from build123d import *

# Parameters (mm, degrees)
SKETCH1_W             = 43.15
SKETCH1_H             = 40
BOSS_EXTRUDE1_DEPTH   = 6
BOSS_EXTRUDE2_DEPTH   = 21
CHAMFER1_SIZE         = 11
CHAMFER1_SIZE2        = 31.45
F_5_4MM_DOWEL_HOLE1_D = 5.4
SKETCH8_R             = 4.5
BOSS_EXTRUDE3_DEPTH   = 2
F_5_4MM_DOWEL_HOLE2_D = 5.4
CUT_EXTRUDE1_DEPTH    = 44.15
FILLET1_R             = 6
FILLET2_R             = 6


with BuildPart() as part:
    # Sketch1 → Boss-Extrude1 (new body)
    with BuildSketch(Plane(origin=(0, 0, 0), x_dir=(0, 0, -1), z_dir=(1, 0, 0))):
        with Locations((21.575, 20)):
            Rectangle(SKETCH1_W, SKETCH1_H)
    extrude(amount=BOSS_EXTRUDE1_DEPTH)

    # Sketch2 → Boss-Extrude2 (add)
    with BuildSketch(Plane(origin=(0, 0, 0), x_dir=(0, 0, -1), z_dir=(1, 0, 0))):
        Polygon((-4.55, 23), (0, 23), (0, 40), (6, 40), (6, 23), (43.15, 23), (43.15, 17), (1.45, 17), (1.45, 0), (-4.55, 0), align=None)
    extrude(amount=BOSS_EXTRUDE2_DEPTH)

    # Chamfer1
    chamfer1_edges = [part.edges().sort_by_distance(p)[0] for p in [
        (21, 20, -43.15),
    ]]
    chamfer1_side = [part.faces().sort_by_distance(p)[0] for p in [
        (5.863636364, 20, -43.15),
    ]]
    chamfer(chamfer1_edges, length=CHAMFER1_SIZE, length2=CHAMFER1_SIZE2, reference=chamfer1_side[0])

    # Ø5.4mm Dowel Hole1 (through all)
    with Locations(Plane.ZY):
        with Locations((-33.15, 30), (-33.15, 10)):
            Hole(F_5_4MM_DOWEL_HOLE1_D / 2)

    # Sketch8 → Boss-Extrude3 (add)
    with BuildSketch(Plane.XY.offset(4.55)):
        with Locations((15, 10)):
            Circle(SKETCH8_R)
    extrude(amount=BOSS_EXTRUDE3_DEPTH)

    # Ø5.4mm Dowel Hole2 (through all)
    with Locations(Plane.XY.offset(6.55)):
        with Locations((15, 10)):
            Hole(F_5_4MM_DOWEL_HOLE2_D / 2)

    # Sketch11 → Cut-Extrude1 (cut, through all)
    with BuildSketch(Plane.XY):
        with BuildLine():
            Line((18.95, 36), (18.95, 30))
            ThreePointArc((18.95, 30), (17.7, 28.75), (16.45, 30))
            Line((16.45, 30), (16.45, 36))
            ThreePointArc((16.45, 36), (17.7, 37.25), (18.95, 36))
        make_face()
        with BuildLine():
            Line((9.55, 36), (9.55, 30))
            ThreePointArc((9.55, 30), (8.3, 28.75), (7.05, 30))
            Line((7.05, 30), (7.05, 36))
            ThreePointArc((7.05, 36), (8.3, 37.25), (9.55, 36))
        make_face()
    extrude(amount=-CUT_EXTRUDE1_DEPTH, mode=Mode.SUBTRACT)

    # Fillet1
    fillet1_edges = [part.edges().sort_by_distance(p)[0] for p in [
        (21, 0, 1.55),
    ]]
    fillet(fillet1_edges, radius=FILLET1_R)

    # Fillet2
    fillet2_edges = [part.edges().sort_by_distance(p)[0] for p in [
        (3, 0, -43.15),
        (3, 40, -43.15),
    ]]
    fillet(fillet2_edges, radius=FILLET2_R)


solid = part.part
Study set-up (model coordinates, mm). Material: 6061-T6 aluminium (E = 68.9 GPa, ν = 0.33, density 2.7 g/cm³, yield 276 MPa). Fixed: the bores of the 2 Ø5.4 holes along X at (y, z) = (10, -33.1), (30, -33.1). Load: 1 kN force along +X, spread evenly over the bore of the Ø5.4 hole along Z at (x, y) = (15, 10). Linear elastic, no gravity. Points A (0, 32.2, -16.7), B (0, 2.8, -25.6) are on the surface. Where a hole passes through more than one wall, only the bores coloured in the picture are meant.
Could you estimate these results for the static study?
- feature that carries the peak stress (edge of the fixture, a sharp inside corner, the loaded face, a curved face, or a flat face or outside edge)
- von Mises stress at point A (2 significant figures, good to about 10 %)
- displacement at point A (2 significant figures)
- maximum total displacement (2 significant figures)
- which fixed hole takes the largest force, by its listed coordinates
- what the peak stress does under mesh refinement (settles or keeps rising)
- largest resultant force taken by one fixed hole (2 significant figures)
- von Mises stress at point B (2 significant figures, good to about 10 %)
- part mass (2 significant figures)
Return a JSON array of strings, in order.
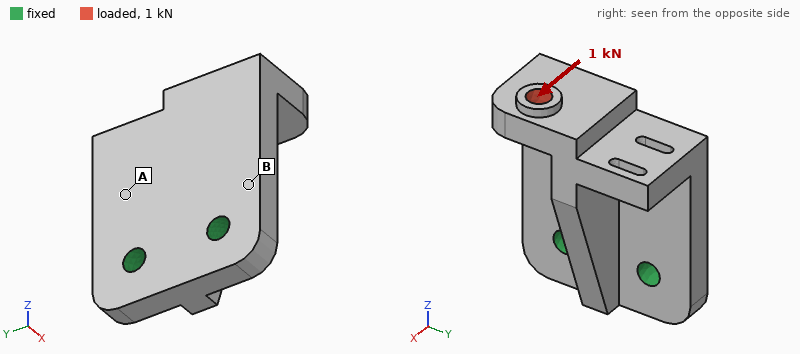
["edge of the fixture", "27 MPa", "0.036 mm", "0.20 mm", "(10, -33.1)", "keeps rising", "970 N", "64 MPa", "45 g"]
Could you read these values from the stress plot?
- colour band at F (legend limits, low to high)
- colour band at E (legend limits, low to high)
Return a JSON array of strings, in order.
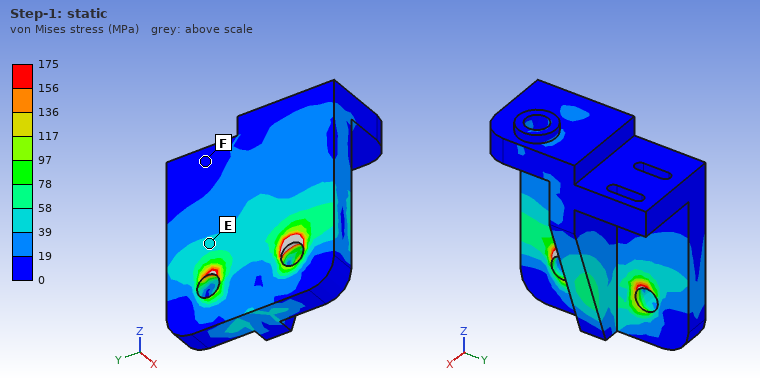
["0 to 19 MPa", "39 to 58 MPa"]
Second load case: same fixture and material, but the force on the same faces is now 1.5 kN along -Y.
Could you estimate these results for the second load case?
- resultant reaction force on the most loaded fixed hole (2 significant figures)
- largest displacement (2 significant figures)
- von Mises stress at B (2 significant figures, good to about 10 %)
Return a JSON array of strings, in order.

["2.5 kN", "0.10 mm", "42 MPa"]
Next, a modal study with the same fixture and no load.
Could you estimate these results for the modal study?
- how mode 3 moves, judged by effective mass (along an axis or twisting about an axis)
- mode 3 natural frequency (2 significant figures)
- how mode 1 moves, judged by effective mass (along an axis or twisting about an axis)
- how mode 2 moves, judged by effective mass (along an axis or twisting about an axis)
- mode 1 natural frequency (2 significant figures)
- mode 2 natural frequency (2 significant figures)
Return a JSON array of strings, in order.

["along Y", "10 kHz", "along X", "along Y", "3300 Hz", "5700 Hz"]
